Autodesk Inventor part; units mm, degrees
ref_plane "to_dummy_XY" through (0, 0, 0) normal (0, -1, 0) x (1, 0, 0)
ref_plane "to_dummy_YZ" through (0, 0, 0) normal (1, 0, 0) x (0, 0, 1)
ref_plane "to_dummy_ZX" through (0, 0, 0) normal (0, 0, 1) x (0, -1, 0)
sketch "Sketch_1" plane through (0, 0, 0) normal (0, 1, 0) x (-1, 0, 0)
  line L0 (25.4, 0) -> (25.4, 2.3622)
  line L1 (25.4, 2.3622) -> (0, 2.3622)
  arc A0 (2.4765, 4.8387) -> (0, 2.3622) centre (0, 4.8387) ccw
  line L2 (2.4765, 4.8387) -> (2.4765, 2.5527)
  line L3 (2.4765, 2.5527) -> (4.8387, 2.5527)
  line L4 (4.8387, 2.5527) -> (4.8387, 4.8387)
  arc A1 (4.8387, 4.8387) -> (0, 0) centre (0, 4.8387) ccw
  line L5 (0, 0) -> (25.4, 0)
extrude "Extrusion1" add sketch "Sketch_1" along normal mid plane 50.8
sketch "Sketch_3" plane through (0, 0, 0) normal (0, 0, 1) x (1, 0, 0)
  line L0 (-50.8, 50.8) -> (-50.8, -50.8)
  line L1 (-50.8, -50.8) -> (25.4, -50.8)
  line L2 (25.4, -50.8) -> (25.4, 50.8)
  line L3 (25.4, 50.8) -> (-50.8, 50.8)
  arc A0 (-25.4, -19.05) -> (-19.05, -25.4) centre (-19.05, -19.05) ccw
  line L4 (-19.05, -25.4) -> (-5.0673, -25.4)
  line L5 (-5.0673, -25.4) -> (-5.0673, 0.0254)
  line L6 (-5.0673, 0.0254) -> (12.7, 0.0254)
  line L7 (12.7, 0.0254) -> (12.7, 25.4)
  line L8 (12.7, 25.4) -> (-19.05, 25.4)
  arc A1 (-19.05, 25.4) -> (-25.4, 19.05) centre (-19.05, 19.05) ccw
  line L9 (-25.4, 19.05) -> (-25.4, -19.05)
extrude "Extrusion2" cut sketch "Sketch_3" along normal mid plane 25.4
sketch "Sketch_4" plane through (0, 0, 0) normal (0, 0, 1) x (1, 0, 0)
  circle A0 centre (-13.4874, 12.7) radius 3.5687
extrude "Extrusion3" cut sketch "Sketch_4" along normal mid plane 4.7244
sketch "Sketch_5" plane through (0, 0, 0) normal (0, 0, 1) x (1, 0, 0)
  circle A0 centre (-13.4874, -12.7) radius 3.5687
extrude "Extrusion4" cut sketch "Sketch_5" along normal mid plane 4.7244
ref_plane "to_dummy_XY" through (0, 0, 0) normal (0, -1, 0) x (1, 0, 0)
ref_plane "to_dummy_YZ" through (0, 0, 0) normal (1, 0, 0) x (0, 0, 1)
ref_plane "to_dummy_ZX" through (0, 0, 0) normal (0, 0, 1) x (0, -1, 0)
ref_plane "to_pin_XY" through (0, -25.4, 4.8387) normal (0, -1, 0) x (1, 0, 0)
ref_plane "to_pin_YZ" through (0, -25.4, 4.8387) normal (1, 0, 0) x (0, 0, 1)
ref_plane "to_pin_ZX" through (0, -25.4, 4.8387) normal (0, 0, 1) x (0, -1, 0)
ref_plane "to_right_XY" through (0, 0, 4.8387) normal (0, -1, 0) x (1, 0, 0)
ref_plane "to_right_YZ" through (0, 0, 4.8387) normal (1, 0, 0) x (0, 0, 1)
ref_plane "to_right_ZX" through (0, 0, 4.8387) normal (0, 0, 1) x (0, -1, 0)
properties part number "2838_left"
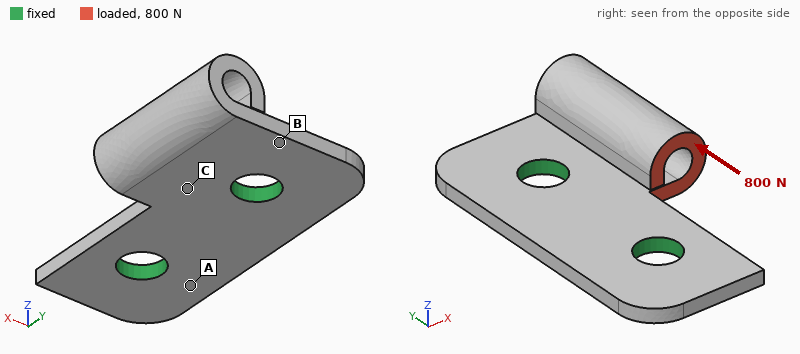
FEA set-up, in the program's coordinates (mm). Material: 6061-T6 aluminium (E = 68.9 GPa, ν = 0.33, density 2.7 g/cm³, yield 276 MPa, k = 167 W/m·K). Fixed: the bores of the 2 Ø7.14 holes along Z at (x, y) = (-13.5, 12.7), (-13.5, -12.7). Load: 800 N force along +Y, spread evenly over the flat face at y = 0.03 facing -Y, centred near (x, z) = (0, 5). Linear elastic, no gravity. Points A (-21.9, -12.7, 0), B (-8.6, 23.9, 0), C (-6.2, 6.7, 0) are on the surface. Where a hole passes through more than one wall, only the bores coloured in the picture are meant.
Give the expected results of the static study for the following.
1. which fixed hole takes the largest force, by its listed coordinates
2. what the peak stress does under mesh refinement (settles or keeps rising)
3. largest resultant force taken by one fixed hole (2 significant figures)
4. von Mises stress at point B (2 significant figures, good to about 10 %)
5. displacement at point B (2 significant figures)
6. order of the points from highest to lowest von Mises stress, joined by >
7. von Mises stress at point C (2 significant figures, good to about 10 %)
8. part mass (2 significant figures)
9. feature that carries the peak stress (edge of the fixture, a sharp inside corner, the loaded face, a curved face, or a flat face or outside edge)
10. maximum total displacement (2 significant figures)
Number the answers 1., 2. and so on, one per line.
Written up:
1. (-13.5, 12.7)
2. keeps rising
3. 660 N
4. 59 MPa
5. 0.034 mm
6. B > C > A
7. 32 MPa
8. 9.9 g
9. a sharp inside corner
10. 0.16 mm
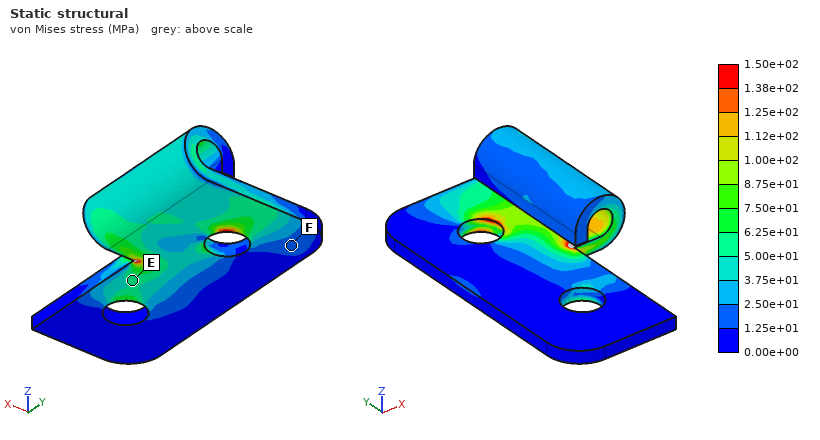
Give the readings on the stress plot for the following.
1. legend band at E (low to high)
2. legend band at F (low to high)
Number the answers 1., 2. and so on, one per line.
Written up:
1. 5.00e+01 to 6.25e+01 MPa
2. 1.25e+01 to 2.50e+01 MPa
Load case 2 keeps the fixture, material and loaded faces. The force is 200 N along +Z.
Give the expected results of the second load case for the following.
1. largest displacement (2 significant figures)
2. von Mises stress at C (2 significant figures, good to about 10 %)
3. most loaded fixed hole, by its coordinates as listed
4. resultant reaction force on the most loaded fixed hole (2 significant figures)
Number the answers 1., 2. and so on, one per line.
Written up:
1. 0.15 mm
2. 59 MPa
3. (-13.5, 12.7)
4. 130 N
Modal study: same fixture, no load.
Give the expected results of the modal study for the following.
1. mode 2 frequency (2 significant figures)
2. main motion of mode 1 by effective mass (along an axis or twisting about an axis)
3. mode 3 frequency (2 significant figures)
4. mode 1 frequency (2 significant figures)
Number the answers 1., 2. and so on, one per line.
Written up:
1. 5400 Hz
2. along Z
3. 7900 Hz
4. 4100 Hz
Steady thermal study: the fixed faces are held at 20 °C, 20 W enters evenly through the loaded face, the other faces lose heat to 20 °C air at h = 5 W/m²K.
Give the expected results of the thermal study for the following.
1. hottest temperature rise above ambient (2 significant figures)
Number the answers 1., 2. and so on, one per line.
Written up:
1. 54 K
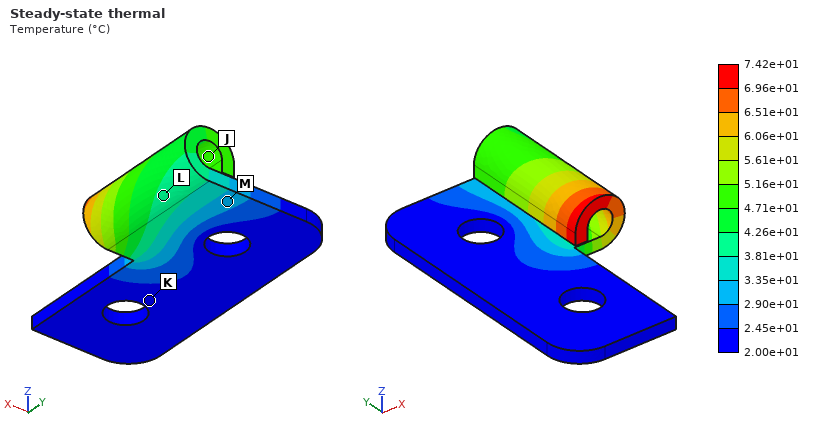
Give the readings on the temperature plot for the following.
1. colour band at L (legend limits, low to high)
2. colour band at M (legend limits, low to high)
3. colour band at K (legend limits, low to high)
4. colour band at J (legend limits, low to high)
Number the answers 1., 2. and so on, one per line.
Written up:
1. 3.81e+01 to 4.26e+01 °C
2. 2.90e+01 to 3.35e+01 °C
3. 2.00e+01 to 2.45e+01 °C
4. 4.71e+01 to 5.16e+01 °C
